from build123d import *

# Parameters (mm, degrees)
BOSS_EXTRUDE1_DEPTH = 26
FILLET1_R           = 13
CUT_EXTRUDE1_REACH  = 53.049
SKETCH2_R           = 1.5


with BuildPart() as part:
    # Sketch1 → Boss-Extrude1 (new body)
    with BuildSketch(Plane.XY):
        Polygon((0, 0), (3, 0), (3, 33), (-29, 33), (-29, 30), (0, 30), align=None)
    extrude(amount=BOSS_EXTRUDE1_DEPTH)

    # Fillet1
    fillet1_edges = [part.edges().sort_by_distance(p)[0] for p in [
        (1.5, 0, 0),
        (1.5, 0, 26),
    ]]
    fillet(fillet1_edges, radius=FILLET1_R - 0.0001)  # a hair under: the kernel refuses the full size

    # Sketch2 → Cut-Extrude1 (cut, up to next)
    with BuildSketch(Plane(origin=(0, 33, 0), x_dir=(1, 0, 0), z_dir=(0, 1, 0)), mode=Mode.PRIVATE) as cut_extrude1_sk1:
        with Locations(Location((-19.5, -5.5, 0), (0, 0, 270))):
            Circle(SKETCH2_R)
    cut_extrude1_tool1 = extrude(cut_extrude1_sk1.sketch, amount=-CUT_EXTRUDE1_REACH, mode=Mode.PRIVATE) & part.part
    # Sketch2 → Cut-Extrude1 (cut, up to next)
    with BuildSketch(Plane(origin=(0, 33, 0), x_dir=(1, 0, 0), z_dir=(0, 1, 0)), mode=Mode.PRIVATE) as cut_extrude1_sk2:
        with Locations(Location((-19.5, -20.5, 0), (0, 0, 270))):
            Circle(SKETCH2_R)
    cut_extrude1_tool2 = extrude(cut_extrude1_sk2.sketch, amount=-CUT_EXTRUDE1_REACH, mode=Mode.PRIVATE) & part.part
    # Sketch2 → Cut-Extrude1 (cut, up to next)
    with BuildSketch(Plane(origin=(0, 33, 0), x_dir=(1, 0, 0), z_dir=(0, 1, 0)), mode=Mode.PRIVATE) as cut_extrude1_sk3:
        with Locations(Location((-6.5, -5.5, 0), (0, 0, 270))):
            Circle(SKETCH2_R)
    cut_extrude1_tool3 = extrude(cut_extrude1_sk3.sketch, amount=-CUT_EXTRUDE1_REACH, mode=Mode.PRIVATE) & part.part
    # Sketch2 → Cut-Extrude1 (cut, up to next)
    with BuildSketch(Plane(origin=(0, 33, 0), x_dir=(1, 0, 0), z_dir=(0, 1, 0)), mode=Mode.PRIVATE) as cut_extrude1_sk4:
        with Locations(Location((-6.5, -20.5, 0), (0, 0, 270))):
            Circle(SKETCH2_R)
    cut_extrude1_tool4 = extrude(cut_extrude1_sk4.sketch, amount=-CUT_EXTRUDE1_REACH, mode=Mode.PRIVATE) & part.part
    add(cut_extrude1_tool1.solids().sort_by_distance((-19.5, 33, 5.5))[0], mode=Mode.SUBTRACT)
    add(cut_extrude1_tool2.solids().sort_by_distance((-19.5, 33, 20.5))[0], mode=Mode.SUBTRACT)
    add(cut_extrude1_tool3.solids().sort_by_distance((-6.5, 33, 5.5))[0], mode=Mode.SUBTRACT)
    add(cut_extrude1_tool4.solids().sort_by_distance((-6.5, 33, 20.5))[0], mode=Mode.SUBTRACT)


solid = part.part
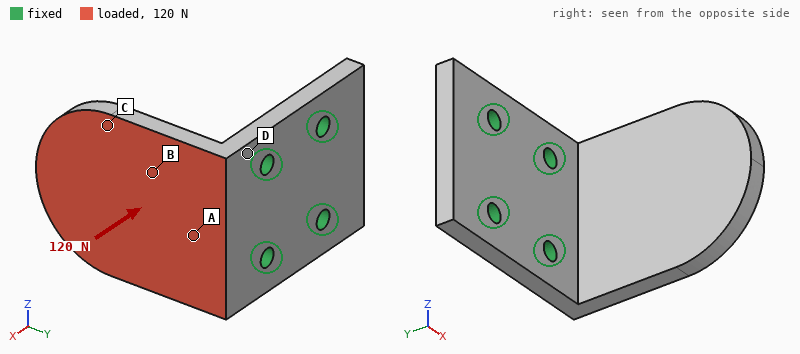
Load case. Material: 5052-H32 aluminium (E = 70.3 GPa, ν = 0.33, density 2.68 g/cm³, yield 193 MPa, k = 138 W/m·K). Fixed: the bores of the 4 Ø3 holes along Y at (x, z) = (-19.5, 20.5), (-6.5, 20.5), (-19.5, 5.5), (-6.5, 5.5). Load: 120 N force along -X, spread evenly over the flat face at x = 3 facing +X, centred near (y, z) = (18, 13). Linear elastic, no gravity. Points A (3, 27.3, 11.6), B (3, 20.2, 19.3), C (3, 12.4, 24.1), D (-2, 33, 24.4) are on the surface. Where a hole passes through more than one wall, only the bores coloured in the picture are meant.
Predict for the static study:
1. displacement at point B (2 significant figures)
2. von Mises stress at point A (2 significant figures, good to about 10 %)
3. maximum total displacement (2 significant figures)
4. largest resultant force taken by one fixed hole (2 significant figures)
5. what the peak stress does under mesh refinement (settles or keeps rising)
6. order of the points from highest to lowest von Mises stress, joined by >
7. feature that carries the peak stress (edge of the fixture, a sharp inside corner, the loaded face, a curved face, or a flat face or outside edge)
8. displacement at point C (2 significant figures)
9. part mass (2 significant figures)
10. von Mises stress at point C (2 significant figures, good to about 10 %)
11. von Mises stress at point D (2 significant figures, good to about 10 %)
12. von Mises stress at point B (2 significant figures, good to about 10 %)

0.051 mm
29 MPa
0.17 mm
55 N
keeps rising
D > A > B > C
edge of the fixture
0.094 mm
12 g
5.5 MPa
38 MPa
15 MPa
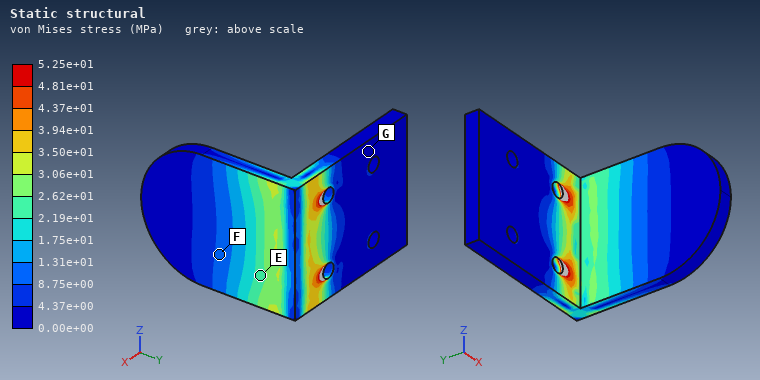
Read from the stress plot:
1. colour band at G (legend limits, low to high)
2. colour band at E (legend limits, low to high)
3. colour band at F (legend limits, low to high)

0.00e+00 to 4.37e+00 MPa
2.19e+01 to 2.62e+01 MPa
8.75e+00 to 1.31e+01 MPa
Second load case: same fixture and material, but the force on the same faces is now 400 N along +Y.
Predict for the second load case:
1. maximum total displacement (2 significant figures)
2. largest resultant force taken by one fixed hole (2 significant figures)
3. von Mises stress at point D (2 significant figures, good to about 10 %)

0.17 mm
230 N
47 MPa
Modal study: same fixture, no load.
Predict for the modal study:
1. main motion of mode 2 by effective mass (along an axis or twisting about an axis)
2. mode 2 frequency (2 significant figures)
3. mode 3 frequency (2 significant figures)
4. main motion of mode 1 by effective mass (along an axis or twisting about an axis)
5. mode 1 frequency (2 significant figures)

along Z
5600 Hz
8600 Hz
along X
2200 Hz
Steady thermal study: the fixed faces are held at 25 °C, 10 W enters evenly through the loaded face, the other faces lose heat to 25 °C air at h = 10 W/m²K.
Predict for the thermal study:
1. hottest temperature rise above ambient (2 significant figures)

19 K
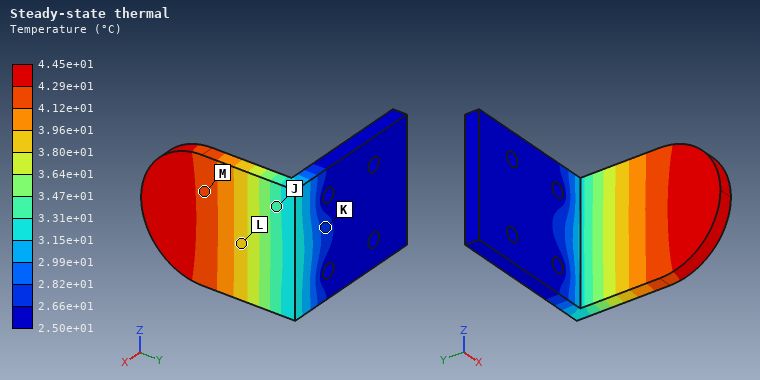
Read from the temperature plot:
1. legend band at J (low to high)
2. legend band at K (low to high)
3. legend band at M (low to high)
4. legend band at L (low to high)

3.31e+01 to 3.47e+01 °C
2.66e+01 to 2.82e+01 °C
4.12e+01 to 4.29e+01 °C
3.80e+01 to 3.96e+01 °C
